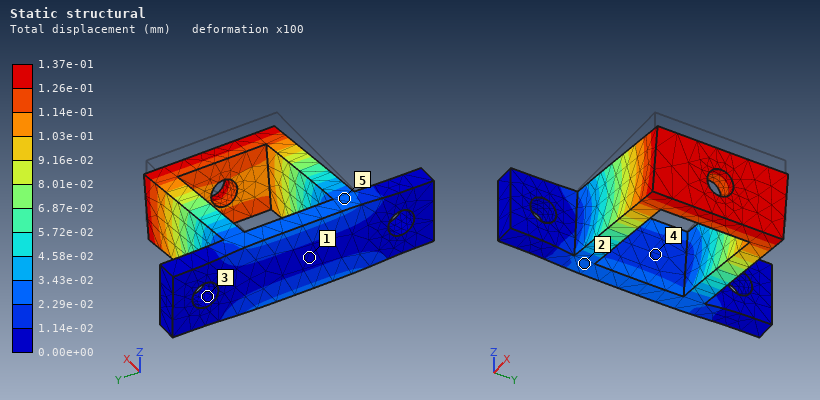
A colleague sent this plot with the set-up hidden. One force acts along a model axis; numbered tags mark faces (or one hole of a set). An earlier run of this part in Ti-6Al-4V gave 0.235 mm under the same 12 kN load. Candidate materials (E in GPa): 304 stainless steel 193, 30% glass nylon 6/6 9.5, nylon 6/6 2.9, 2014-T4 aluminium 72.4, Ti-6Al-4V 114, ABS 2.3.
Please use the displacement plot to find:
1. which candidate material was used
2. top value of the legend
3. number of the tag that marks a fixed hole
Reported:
304 stainless steel
1.37e-01 mm
3
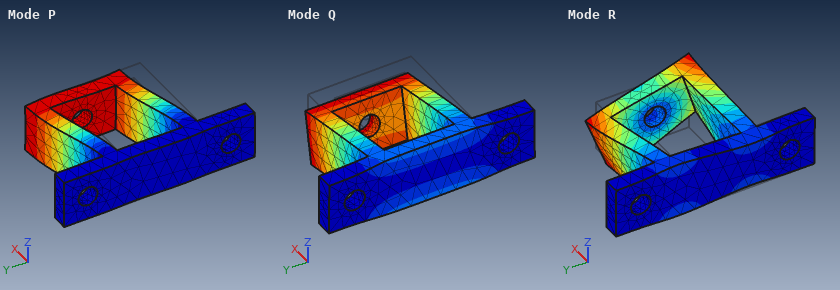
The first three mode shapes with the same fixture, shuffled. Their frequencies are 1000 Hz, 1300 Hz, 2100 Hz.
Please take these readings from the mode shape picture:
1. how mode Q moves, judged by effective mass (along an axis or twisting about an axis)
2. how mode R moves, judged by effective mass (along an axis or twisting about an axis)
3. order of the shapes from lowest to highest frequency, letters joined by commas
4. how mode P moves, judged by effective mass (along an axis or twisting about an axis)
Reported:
along Z
twisting about X
Q, P, R
along Y
